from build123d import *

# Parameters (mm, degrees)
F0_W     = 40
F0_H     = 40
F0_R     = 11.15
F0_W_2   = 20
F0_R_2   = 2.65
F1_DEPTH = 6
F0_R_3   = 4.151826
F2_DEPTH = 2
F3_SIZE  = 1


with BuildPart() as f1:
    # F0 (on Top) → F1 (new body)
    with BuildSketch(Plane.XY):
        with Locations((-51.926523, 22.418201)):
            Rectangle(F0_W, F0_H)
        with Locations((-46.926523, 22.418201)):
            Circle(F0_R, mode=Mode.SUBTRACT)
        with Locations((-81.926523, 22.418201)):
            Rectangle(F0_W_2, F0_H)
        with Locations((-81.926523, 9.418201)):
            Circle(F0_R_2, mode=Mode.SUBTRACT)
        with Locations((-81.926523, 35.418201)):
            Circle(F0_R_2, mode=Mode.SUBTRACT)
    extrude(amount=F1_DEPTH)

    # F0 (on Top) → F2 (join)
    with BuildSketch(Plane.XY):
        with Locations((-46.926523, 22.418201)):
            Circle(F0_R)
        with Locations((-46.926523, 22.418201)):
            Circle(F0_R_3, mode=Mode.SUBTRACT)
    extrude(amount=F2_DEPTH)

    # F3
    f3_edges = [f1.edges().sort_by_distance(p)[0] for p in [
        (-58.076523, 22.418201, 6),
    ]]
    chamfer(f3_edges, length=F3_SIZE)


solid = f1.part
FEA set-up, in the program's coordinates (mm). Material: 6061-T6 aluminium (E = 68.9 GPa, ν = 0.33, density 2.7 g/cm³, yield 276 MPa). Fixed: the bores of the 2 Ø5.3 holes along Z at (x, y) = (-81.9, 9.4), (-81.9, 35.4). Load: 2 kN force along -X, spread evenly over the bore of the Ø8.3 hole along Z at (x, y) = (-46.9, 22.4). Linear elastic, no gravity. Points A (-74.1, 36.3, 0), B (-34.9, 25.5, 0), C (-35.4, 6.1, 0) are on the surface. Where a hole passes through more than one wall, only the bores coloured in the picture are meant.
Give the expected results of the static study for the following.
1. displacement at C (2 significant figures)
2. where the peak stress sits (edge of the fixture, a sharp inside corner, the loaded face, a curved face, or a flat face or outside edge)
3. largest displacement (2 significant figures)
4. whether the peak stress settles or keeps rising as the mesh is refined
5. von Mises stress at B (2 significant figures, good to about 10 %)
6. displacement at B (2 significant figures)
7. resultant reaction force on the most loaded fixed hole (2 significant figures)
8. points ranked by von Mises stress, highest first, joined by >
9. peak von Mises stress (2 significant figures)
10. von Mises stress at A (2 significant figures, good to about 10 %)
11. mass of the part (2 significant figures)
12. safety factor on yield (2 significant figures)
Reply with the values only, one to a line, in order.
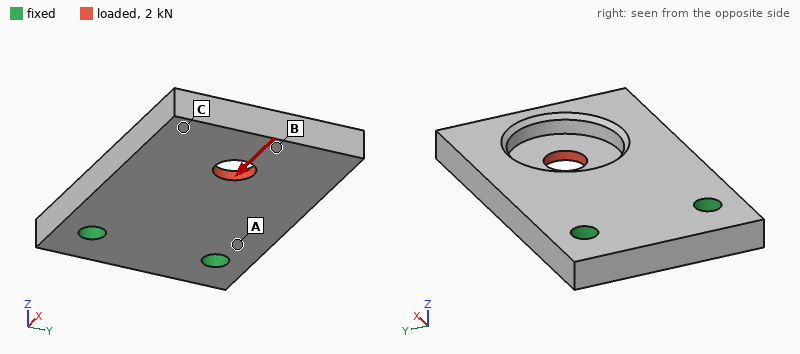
74 µm
the loaded face
85 µm
settles
16 MPa
77 µm
1.0 kN
A > B > C
80 MPa
29 MPa
34 g
3.4
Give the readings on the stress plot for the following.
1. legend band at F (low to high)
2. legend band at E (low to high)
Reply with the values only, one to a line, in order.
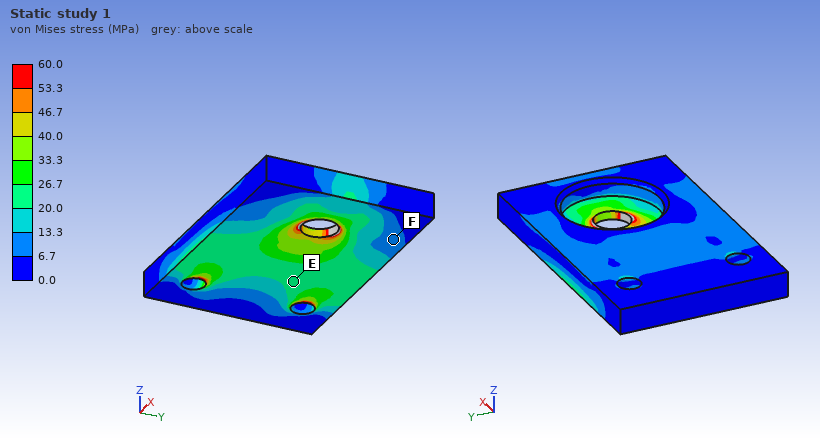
6.7 to 13.3 MPa
20.0 to 26.7 MPa
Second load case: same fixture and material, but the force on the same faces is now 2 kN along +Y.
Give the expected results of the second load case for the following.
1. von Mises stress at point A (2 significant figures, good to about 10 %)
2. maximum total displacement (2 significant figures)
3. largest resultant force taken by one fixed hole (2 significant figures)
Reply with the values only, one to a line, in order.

27 MPa
53 µm
2.6 kN
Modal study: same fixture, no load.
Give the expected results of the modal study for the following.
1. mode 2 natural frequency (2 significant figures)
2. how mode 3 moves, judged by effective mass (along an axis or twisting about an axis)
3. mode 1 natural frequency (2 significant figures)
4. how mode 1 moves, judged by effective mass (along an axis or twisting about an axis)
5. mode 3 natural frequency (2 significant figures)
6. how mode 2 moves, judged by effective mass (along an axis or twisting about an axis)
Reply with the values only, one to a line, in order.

4900 Hz
along Y
2200 Hz
along Z
9400 Hz
twisting about X
